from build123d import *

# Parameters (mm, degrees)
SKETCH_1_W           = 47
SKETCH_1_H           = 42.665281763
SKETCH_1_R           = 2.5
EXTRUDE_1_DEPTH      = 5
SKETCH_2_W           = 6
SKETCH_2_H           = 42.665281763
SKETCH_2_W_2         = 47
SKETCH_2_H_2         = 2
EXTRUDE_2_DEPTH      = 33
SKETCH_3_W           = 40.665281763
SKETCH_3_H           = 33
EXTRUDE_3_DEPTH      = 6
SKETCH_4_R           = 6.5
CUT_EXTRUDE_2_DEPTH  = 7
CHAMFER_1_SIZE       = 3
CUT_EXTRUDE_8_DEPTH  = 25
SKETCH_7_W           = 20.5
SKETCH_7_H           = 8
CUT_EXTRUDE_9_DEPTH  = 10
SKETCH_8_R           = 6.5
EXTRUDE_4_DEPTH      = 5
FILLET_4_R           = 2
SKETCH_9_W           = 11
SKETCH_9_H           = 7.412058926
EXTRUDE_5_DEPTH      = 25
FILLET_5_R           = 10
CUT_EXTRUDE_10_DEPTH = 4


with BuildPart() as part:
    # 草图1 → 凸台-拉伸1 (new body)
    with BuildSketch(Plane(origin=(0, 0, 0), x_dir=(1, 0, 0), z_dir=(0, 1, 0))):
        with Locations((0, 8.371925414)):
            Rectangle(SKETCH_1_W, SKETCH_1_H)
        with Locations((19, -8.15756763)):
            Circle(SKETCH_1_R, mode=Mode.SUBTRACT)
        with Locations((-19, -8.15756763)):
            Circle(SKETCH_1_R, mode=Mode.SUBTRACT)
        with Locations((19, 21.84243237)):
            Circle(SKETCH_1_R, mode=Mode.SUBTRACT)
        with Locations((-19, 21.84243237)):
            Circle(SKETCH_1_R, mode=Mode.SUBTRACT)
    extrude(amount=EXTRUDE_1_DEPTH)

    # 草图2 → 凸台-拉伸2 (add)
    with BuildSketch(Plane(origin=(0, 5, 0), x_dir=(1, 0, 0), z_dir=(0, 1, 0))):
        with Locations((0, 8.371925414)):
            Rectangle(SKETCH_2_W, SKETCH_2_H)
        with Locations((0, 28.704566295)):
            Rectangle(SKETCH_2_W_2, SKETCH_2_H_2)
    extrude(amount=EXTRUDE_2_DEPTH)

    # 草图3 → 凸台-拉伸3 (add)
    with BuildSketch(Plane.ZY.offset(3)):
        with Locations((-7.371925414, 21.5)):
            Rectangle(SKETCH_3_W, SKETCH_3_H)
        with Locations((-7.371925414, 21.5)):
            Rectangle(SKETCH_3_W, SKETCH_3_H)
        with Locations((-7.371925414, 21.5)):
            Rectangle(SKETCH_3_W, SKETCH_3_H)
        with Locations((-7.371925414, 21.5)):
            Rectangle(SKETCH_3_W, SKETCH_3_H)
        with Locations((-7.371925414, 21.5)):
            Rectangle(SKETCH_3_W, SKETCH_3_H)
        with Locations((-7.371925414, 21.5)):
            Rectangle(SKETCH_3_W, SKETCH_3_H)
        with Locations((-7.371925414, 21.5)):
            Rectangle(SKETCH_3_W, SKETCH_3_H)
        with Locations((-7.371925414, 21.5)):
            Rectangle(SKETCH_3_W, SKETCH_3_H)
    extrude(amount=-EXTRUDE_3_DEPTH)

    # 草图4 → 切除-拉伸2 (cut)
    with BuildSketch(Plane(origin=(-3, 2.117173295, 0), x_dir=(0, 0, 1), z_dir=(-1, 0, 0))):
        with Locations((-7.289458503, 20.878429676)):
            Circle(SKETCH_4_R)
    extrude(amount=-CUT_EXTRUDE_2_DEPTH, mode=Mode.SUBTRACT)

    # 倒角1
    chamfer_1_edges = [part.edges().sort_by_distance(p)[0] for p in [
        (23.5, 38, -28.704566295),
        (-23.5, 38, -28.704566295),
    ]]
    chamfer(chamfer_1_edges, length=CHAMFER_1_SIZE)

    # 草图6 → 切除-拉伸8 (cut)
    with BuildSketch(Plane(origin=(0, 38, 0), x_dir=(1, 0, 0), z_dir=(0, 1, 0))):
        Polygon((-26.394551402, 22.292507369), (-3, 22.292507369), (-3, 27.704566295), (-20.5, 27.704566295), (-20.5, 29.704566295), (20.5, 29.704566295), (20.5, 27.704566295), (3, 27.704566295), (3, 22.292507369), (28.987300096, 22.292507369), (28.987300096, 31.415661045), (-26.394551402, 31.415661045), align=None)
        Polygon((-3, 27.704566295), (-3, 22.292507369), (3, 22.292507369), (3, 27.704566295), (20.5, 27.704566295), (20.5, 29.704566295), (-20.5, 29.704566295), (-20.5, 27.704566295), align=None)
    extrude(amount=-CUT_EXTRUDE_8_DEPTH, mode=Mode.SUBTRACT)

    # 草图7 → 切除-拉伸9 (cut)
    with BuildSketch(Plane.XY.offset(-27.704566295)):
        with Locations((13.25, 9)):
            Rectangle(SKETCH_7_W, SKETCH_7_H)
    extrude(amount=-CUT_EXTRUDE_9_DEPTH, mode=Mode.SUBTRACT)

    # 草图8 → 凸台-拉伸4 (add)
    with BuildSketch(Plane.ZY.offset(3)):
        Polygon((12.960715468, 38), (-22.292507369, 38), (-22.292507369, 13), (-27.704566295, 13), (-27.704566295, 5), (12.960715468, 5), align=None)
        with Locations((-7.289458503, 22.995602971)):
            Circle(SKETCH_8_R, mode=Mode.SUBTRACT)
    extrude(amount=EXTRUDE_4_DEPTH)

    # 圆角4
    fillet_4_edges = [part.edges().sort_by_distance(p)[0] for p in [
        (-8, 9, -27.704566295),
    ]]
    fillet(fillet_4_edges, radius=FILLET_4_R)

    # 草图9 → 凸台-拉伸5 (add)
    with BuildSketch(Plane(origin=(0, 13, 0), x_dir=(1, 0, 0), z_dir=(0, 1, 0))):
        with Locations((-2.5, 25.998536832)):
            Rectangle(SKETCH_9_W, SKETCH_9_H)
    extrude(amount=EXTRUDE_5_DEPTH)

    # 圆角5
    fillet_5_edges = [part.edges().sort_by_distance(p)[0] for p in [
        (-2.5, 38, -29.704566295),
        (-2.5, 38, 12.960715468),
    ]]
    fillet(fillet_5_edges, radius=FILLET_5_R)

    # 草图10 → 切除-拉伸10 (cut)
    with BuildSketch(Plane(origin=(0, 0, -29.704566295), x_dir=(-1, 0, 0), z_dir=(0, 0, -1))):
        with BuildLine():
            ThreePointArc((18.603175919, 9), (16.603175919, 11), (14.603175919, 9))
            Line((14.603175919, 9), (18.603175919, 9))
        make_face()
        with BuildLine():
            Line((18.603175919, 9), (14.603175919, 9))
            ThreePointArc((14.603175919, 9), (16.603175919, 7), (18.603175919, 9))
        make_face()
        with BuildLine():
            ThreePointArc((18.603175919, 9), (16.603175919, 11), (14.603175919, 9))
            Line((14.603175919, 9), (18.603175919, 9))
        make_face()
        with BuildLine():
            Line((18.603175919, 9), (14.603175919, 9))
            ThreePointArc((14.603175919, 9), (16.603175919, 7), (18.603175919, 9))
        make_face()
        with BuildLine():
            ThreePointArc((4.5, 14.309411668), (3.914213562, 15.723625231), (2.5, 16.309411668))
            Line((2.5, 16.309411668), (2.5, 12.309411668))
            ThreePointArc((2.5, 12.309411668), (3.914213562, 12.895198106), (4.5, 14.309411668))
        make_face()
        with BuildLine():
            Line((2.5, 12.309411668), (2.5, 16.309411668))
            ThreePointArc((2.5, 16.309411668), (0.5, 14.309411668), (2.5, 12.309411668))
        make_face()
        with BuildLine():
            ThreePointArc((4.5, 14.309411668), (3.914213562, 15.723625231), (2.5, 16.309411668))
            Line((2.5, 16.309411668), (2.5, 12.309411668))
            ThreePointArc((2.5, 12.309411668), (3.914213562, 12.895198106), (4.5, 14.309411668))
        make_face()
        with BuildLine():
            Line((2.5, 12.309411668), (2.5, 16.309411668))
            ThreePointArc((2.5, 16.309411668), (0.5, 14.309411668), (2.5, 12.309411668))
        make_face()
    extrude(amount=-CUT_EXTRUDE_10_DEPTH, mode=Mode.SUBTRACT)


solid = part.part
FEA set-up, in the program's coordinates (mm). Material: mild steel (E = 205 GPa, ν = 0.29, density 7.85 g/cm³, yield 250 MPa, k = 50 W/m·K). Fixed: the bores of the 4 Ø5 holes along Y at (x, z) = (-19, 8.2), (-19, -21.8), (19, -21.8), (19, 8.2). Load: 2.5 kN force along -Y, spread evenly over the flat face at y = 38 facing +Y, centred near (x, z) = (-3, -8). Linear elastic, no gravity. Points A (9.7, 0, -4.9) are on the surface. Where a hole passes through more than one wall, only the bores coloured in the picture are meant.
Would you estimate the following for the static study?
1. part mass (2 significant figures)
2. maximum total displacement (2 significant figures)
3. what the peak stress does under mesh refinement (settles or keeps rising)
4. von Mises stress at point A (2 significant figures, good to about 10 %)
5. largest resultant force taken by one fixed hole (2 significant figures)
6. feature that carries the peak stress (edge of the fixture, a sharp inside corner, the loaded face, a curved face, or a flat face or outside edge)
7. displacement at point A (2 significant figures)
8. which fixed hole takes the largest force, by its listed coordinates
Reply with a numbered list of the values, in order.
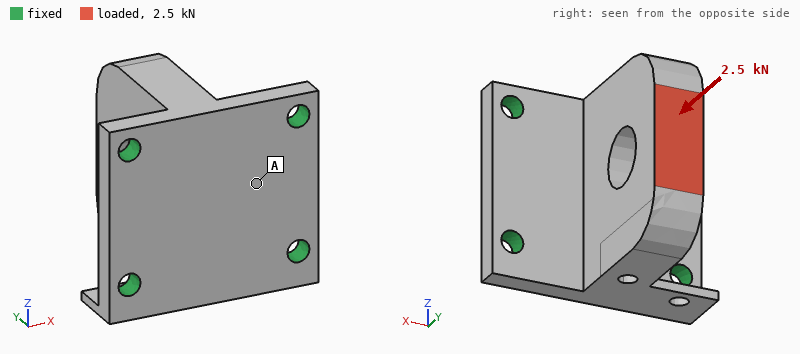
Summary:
1. 180 g
2. 10 µm
3. keeps rising
4. 10 MPa
5. 800 N
6. edge of the fixture
7. 4.4 µm
8. (-19, -21.8)
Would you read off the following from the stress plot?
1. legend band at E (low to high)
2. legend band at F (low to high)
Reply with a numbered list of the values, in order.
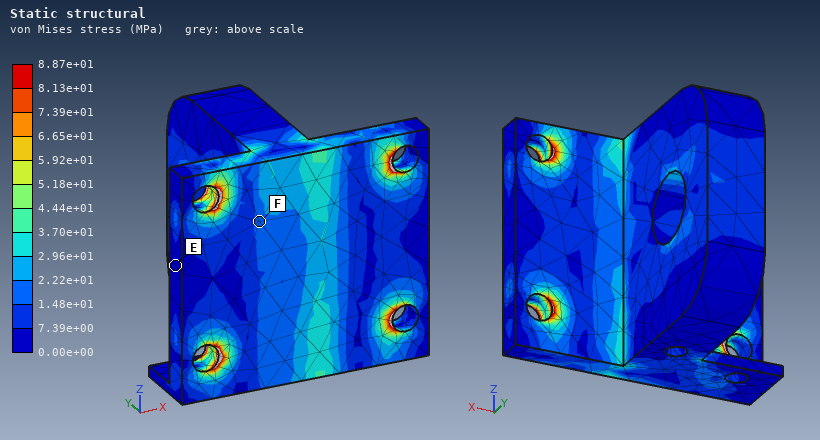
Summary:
1. 0.00e+00 to 7.39e+00 MPa
2. 1.48e+01 to 2.22e+01 MPa
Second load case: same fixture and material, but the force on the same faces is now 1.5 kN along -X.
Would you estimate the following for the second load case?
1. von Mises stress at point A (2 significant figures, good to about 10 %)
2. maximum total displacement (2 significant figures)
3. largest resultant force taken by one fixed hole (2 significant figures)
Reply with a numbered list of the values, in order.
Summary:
1. 28 MPa
2. 54 µm
3. 1.1 kN
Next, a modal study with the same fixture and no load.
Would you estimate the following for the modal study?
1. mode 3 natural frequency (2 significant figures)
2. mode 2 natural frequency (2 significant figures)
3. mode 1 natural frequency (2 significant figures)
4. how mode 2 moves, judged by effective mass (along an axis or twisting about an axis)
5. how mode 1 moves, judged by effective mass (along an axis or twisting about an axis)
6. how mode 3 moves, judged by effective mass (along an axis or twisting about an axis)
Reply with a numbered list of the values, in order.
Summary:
1. 9300 Hz
2. 6000 Hz
3. 4900 Hz
4. along Z
5. along X
6. along Y
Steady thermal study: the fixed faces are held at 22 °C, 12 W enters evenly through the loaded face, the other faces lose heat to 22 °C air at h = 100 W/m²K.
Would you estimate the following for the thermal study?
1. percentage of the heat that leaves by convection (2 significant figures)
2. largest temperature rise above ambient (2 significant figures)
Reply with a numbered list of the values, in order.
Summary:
1. 48 %
2. 26 K
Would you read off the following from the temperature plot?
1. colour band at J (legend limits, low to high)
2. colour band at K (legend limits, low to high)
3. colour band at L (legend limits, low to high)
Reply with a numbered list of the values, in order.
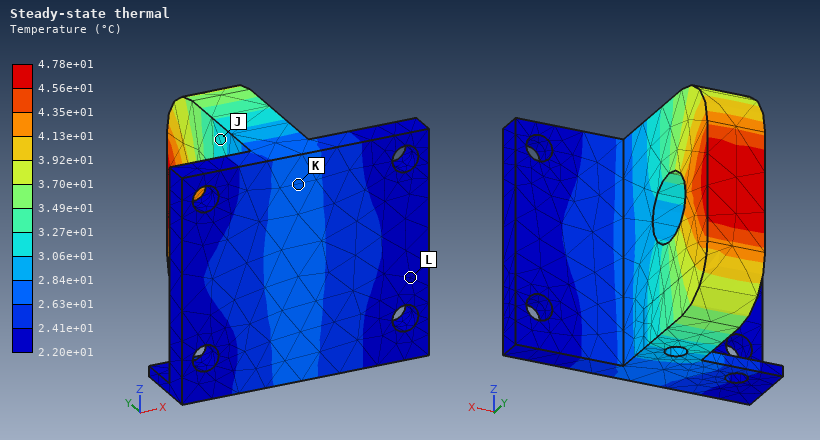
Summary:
1. 3.06e+01 to 3.27e+01 °C
2. 2.63e+01 to 2.84e+01 °C
3. 2.20e+01 to 2.41e+01 °C
